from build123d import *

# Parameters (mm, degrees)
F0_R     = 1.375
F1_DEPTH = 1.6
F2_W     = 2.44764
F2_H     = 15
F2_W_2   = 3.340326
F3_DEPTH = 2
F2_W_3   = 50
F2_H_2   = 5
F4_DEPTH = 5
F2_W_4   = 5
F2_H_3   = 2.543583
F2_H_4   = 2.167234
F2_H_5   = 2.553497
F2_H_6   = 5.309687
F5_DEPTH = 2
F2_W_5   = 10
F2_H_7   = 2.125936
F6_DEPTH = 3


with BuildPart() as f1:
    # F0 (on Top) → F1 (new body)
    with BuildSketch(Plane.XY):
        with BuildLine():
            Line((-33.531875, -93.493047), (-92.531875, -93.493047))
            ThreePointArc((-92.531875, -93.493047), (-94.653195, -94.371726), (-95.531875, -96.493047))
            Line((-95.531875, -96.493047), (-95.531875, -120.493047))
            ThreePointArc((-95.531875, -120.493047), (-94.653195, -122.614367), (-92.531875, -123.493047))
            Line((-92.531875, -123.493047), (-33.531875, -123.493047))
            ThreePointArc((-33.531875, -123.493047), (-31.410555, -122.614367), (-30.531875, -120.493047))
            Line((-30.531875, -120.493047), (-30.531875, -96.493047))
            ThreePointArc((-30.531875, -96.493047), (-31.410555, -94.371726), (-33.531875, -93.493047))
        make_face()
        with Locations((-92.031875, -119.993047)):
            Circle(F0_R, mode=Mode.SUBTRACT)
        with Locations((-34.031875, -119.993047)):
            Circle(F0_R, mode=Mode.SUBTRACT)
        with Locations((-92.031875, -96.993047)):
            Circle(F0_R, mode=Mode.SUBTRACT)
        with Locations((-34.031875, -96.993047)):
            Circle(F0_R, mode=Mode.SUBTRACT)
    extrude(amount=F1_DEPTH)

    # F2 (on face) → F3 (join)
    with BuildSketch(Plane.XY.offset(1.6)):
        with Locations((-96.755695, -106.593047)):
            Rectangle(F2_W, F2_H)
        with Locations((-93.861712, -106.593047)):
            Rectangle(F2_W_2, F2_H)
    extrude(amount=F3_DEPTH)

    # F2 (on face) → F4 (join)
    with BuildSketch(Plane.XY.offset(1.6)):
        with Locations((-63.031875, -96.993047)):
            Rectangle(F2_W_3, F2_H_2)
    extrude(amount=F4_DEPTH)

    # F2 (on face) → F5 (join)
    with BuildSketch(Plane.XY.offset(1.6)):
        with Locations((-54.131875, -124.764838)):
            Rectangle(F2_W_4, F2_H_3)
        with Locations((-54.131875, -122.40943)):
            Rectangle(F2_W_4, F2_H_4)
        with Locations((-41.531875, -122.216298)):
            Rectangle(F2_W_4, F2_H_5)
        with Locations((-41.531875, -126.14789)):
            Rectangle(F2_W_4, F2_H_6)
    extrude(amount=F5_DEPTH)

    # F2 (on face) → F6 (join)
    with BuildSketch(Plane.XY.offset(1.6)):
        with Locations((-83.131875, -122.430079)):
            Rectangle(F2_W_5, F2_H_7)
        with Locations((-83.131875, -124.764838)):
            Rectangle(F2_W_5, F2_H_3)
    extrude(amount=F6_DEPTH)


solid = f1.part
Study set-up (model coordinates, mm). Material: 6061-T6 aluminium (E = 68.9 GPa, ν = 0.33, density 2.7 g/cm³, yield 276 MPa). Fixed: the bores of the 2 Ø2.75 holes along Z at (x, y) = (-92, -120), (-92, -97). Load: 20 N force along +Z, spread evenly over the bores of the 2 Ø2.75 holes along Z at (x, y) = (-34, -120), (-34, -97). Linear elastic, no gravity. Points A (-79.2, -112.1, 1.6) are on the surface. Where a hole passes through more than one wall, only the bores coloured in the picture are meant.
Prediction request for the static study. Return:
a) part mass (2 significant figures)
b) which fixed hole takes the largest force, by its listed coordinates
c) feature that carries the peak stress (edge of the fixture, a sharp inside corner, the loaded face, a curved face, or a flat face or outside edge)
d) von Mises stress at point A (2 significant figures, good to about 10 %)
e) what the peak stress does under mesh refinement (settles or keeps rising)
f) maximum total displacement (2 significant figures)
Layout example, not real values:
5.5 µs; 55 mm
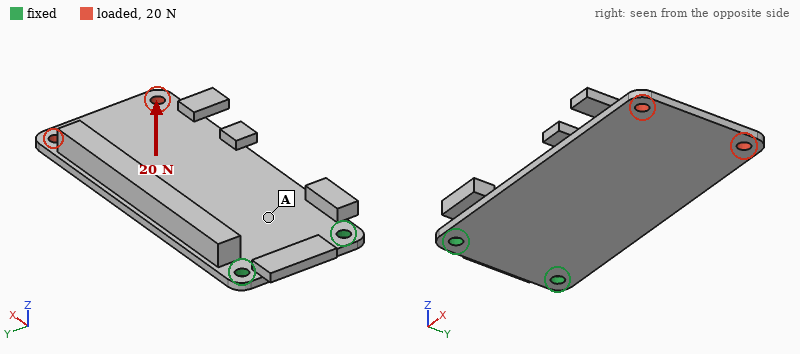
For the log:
13 g; (-92, -120); edge of the fixture; 19 MPa; keeps rising; 0.78 mm
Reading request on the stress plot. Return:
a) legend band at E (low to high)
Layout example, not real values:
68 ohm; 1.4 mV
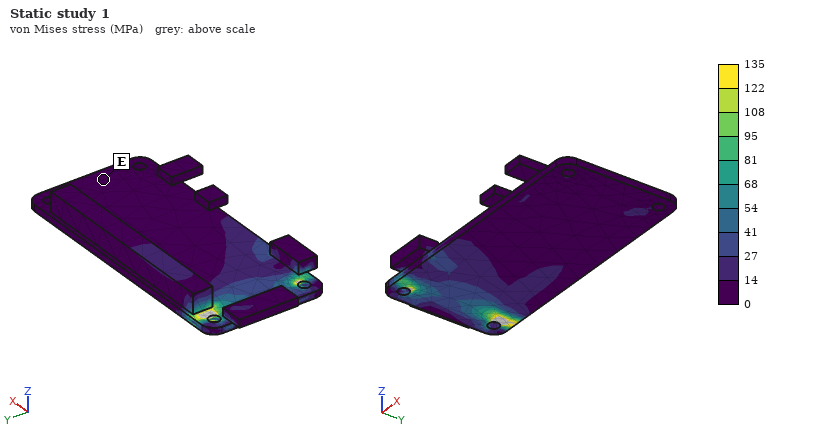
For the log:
0 to 14 MPa
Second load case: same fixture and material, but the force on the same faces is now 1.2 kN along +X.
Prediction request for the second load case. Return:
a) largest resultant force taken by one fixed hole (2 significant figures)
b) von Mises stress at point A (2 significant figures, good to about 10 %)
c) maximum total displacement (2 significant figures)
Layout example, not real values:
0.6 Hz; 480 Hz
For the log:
610 N; 16 MPa; 0.13 mm
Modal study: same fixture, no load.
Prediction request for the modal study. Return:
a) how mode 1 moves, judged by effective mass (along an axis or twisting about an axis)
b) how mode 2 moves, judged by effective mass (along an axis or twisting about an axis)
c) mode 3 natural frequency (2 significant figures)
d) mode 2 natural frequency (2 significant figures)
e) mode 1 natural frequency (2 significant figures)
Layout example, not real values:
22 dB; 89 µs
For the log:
along Z; twisting about X; 3600 Hz; 1700 Hz; 440 Hz
